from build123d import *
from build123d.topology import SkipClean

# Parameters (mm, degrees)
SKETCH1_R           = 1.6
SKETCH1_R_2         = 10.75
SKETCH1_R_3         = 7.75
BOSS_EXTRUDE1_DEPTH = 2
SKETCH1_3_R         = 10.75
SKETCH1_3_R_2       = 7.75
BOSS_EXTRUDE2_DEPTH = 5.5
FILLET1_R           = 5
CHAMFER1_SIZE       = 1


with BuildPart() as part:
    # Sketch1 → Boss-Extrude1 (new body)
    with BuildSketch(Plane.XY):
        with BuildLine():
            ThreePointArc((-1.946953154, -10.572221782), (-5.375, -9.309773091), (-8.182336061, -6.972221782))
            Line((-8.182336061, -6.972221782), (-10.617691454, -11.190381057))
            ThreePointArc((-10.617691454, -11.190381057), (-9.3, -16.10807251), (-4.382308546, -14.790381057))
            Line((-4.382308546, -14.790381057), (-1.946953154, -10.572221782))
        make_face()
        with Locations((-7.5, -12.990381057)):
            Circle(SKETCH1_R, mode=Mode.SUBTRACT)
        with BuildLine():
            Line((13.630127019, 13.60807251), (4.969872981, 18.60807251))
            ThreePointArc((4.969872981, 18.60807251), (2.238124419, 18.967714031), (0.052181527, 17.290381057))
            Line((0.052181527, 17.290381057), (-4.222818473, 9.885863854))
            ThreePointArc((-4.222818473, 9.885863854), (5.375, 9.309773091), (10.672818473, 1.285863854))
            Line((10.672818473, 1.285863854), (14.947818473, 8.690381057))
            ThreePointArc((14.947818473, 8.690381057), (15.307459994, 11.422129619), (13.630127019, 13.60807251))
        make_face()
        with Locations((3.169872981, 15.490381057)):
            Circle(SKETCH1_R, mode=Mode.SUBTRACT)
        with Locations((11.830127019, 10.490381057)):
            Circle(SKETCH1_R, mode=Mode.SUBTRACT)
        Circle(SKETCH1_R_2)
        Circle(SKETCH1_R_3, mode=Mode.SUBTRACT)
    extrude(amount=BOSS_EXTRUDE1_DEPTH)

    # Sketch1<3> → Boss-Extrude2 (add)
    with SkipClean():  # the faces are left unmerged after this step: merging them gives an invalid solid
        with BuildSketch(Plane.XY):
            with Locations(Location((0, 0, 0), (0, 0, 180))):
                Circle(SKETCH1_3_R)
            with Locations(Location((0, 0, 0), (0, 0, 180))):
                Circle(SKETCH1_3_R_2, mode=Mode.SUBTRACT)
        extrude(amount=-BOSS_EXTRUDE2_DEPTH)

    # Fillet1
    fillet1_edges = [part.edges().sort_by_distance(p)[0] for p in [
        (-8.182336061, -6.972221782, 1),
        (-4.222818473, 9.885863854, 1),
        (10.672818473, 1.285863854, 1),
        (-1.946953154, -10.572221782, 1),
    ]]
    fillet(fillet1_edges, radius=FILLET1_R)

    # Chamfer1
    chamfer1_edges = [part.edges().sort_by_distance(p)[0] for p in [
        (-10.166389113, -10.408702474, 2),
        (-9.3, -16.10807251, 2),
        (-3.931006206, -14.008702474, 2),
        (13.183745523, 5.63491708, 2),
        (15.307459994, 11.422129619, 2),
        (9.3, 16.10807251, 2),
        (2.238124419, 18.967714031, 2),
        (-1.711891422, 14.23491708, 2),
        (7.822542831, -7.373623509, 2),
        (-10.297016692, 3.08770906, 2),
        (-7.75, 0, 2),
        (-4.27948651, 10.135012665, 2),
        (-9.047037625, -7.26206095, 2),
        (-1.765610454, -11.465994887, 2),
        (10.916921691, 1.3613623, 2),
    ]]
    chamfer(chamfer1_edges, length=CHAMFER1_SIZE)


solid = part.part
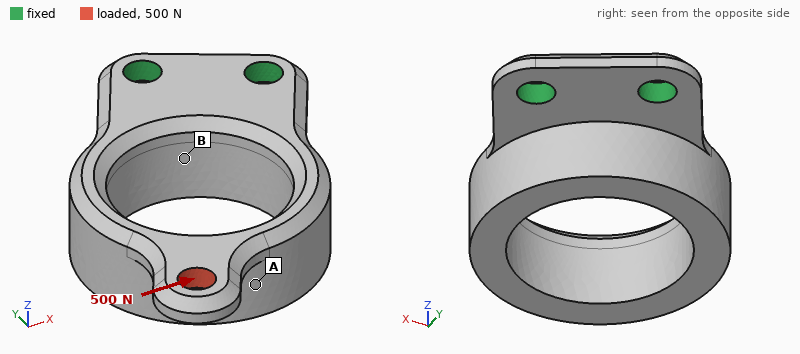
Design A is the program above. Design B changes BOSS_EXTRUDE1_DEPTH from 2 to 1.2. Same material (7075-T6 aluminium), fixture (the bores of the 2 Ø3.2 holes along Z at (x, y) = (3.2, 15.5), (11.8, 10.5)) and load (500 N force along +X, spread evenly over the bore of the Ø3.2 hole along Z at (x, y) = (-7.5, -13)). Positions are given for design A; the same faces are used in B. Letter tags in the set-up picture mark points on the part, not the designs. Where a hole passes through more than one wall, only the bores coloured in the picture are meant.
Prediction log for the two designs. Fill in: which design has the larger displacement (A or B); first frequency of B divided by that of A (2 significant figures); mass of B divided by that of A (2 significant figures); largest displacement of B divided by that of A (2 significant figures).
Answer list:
B
0.57
0.82
1.5
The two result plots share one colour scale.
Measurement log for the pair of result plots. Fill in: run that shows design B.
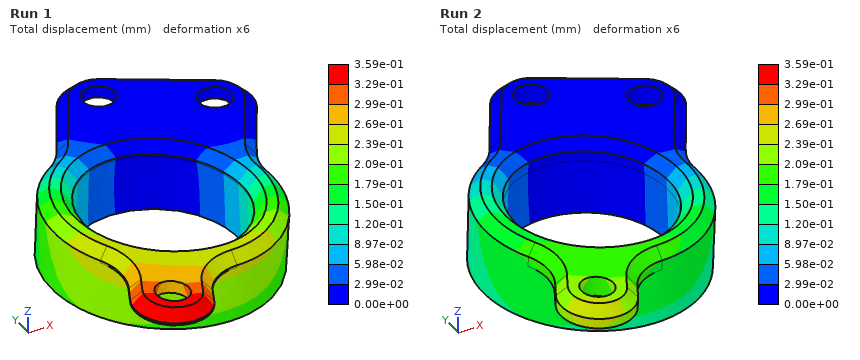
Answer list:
Run 1
